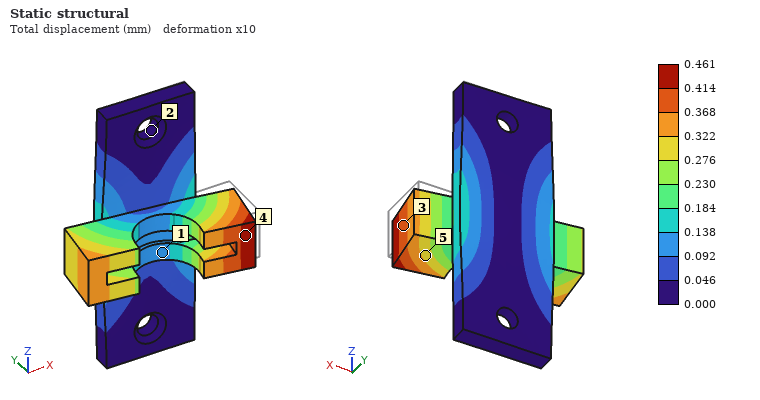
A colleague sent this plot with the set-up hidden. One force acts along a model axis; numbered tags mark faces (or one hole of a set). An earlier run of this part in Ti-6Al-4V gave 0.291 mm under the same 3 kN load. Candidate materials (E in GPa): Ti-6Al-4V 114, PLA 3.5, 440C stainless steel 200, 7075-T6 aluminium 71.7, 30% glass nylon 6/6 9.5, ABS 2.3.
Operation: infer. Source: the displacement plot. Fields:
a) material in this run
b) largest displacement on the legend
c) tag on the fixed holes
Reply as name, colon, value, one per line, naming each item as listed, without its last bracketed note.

material in this run: 7075-T6 aluminium
largest displacement on the legend: 0.461 mm
tag on the fixed holes: 2
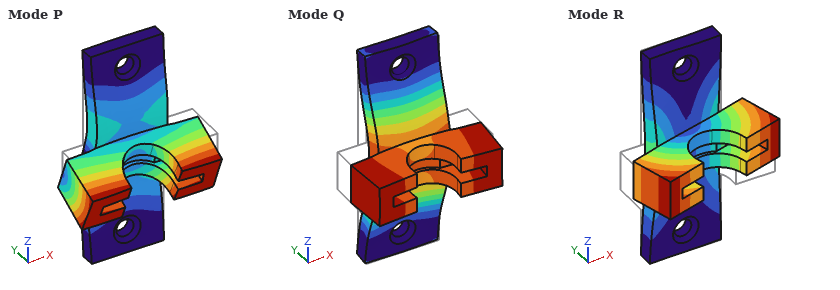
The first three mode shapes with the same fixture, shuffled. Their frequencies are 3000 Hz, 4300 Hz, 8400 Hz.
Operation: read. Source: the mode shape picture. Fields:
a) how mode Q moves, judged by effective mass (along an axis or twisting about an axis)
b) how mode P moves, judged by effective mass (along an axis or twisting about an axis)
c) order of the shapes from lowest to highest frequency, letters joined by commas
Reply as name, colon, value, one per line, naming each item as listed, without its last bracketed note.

how mode Q moves, judged by effective mass: along Y
how mode P moves, judged by effective mass: along Z
order of the shapes from lowest to highest frequency, letters joined by commas: R, Q, P
